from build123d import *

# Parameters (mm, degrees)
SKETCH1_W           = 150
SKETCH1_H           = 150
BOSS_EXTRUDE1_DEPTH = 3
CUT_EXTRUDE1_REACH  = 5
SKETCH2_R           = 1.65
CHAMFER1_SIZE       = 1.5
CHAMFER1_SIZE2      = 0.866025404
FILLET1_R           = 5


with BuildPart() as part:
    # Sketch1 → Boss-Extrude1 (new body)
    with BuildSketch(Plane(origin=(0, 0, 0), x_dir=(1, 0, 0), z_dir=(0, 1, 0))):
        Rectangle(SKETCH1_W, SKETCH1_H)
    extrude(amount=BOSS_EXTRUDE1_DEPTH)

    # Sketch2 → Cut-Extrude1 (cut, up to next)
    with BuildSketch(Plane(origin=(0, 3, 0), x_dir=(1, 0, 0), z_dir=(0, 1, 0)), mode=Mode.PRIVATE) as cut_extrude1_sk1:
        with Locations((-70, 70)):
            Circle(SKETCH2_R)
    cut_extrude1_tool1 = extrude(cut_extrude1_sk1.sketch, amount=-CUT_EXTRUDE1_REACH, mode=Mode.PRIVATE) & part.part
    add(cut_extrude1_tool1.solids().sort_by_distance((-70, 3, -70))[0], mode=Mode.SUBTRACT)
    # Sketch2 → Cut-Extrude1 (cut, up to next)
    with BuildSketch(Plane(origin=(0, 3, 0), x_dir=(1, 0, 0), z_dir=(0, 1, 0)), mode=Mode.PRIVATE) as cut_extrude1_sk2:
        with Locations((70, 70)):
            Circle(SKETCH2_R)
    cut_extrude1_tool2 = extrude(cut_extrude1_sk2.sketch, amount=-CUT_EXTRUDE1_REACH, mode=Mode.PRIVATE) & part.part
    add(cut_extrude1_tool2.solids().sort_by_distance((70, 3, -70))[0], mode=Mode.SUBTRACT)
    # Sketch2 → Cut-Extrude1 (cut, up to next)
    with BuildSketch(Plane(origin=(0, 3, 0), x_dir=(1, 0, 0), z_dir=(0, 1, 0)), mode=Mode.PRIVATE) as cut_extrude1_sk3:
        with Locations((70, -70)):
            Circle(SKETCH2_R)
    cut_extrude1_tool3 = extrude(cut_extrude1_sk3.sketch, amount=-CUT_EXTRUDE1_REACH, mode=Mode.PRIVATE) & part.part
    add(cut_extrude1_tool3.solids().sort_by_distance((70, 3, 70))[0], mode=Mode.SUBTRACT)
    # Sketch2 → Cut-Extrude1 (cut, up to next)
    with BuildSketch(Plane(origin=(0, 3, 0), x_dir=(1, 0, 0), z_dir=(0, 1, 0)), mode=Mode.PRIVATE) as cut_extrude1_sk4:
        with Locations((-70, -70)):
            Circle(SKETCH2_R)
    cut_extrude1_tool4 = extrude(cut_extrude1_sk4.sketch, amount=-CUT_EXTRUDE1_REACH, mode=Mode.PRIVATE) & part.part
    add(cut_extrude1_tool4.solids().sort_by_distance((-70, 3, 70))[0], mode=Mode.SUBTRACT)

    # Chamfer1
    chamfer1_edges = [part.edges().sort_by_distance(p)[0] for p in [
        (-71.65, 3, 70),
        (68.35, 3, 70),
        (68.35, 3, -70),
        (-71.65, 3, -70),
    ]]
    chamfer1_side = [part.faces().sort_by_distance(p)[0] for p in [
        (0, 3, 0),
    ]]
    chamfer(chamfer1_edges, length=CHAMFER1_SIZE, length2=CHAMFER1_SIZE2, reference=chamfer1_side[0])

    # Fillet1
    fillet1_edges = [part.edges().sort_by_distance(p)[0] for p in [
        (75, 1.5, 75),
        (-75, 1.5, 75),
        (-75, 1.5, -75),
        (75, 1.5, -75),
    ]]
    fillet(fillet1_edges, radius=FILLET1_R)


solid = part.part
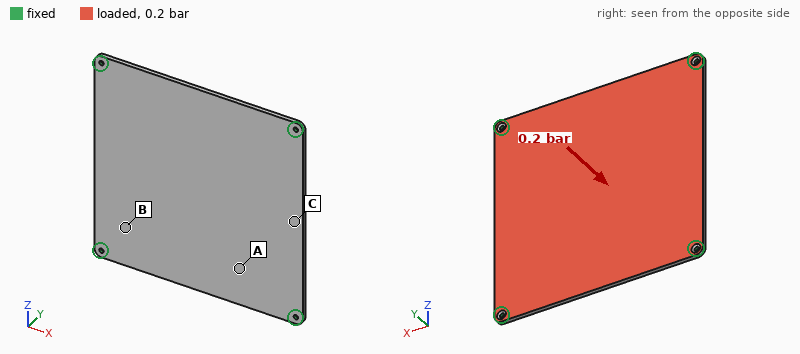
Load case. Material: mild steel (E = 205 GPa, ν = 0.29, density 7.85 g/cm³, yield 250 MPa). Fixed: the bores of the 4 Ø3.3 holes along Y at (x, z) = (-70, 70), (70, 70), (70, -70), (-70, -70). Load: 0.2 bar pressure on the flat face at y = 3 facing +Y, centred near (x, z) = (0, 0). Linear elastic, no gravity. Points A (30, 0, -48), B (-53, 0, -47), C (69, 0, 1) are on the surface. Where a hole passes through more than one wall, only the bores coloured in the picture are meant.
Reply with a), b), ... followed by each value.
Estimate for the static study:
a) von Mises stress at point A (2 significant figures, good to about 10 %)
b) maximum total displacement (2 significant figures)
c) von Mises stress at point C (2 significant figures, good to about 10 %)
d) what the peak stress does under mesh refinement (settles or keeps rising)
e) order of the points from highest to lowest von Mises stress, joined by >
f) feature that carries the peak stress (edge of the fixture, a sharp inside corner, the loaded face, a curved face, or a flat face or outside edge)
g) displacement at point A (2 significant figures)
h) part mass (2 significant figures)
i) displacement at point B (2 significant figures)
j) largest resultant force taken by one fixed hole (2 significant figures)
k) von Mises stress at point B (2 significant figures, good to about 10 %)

a) 12 MPa
b) 0.16 mm
c) 19 MPa
d) keeps rising
e) C > A > B
f) edge of the fixture
g) 0.10 mm
h) 530 g
i) 0.064 mm
j) 150 N
k) 5.8 MPa
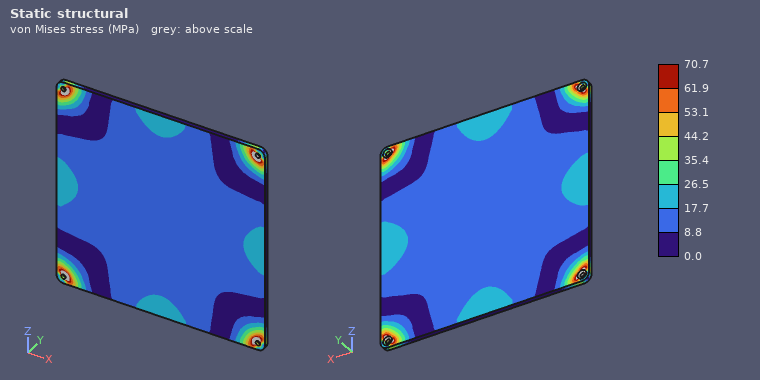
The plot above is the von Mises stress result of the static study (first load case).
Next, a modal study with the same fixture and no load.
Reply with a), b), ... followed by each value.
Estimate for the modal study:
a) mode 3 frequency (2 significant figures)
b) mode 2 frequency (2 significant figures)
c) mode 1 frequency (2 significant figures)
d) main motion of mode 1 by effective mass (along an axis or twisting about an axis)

a) 810 Hz
b) 810 Hz
c) 430 Hz
d) along Y
